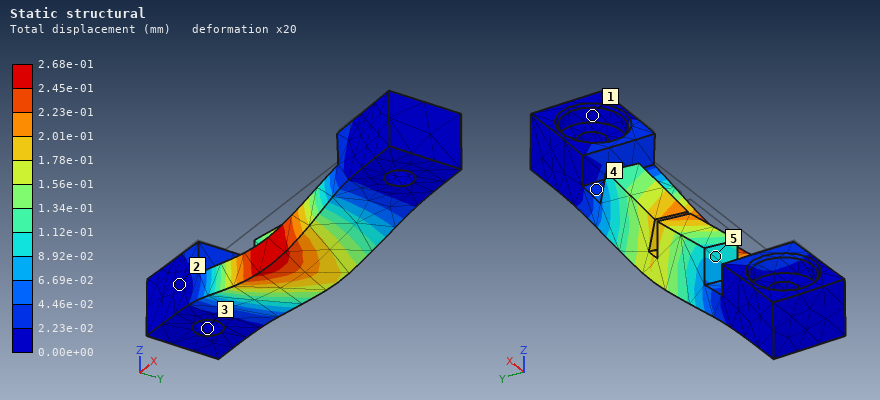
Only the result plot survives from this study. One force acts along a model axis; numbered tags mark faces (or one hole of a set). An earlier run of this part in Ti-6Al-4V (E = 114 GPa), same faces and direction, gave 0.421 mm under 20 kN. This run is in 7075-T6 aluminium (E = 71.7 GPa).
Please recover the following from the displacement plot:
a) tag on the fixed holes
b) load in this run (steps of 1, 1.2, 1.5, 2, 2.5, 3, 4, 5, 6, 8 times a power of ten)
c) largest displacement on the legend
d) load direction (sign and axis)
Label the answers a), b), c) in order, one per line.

a) 3
b) 8 kN
c) 2.68e-01 mm
d) -Z
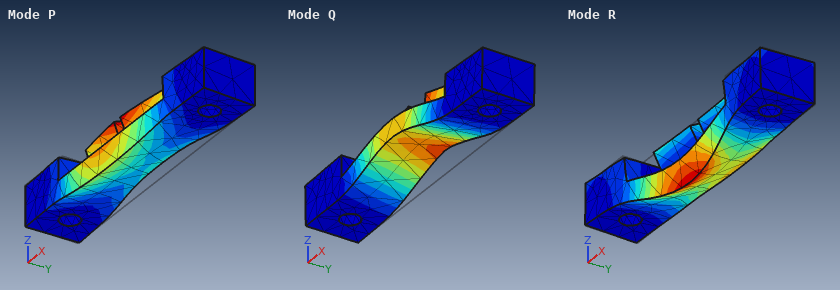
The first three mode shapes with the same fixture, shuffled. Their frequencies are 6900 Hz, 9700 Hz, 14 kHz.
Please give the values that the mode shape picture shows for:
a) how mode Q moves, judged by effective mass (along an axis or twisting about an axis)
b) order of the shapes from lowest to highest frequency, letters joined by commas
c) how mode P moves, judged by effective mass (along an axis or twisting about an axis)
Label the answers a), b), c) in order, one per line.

a) along Z
b) Q, P, R
c) along Y
